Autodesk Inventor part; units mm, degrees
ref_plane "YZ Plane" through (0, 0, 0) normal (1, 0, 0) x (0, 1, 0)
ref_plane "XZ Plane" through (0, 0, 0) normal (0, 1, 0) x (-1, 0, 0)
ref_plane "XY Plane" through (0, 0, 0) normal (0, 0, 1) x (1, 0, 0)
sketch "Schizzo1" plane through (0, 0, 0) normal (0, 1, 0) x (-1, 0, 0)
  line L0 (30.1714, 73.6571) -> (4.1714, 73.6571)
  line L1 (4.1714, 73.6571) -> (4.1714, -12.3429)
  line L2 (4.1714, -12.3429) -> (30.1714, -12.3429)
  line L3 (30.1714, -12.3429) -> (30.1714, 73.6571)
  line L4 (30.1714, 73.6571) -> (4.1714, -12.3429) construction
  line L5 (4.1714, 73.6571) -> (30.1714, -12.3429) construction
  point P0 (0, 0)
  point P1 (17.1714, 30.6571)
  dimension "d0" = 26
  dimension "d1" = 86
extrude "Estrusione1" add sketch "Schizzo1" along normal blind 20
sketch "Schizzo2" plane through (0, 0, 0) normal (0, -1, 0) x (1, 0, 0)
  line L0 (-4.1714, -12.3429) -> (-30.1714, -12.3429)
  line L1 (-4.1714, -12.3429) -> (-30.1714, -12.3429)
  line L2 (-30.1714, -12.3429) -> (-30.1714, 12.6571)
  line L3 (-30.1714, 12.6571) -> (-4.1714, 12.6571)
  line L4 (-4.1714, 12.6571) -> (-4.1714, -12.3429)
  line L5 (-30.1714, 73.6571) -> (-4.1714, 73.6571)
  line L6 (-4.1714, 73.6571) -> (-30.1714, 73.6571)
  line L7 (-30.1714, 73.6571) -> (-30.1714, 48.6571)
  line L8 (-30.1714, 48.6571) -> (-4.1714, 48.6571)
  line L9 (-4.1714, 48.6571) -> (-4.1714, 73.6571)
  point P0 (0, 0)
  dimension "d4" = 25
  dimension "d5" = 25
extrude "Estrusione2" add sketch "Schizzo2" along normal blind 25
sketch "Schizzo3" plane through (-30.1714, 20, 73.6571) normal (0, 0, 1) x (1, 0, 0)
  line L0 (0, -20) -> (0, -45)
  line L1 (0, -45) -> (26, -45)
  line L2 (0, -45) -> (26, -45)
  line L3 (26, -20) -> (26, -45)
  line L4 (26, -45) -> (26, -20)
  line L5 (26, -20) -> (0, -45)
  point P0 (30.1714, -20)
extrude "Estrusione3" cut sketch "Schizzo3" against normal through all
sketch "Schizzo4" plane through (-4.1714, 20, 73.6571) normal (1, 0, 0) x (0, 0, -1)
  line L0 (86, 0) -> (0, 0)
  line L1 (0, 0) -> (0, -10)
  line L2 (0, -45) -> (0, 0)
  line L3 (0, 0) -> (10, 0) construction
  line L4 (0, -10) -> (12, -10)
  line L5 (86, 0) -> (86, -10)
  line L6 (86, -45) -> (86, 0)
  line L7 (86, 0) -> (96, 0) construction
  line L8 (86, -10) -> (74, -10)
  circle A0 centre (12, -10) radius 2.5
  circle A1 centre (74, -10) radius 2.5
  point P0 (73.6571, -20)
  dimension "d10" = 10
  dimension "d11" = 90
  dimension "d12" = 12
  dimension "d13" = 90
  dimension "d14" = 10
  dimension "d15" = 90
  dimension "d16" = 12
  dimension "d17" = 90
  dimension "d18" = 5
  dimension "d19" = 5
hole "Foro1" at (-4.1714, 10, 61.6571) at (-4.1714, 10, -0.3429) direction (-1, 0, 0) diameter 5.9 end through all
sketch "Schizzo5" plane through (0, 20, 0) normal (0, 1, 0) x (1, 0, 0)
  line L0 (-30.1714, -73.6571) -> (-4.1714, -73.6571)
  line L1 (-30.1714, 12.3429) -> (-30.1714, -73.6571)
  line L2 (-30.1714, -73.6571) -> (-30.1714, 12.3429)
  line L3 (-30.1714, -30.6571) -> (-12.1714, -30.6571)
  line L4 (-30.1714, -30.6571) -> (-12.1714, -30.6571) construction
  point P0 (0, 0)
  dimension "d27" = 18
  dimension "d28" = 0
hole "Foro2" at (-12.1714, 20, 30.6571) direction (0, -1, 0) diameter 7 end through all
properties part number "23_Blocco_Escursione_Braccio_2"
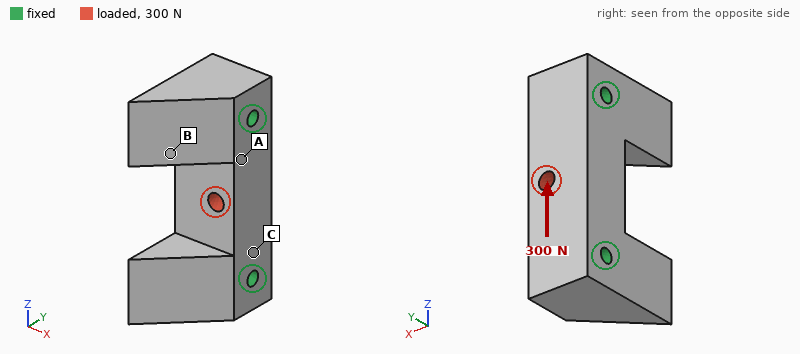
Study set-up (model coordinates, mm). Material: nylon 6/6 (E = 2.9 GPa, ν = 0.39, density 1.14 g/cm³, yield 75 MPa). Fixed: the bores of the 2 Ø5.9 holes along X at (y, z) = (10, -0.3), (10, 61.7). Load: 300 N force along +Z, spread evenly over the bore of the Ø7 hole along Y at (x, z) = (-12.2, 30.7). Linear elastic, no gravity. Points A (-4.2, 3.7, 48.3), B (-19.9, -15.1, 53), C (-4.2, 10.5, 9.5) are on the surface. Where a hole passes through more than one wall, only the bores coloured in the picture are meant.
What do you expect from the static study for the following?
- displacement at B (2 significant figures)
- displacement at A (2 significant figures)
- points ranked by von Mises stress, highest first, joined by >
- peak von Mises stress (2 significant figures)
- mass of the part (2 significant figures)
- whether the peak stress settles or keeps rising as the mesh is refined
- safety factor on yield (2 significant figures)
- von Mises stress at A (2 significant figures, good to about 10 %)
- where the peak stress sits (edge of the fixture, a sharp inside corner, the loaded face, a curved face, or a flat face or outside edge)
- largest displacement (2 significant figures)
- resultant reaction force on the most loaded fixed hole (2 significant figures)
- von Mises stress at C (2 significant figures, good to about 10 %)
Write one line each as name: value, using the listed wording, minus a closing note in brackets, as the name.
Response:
displacement at B: 1.5 µm
displacement at A: 2.0 µm
points ranked by von Mises stress, highest first, joined by >: C > A > B
peak von Mises stress: 1.2 MPa
mass of the part: 67 g
whether the peak stress settles or keeps rising as the mesh is refined: settles
safety factor on yield: 63
von Mises stress at A: 0.38 MPa
where the peak stress sits: the loaded face
largest displacement: 4.8 µm
resultant reaction force on the most loaded fixed hole: 150 N
von Mises stress at C: 0.49 MPa
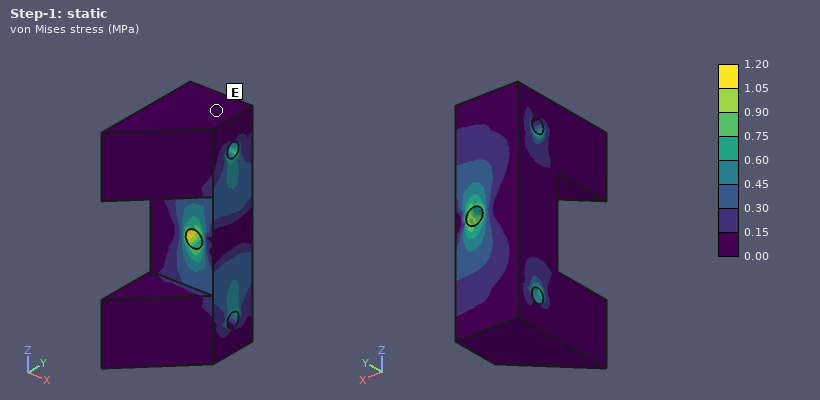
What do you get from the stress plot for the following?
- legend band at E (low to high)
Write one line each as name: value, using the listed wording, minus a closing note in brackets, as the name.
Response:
legend band at E: 0.00 to 0.15 MPa
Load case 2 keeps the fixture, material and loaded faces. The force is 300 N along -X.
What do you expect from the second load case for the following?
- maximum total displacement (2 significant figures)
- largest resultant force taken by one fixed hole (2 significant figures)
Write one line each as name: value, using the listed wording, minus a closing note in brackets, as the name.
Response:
maximum total displacement: 16 µm
largest resultant force taken by one fixed hole: 150 N
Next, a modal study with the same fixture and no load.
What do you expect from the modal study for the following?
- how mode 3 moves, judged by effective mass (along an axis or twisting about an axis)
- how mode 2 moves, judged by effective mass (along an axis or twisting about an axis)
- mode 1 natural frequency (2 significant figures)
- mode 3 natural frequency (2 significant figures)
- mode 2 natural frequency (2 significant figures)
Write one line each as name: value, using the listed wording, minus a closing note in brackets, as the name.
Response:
how mode 3 moves, judged by effective mass: along X
how mode 2 moves, judged by effective mass: along Z
mode 1 natural frequency: 3500 Hz
mode 3 natural frequency: 5500 Hz
mode 2 natural frequency: 5300 Hz
